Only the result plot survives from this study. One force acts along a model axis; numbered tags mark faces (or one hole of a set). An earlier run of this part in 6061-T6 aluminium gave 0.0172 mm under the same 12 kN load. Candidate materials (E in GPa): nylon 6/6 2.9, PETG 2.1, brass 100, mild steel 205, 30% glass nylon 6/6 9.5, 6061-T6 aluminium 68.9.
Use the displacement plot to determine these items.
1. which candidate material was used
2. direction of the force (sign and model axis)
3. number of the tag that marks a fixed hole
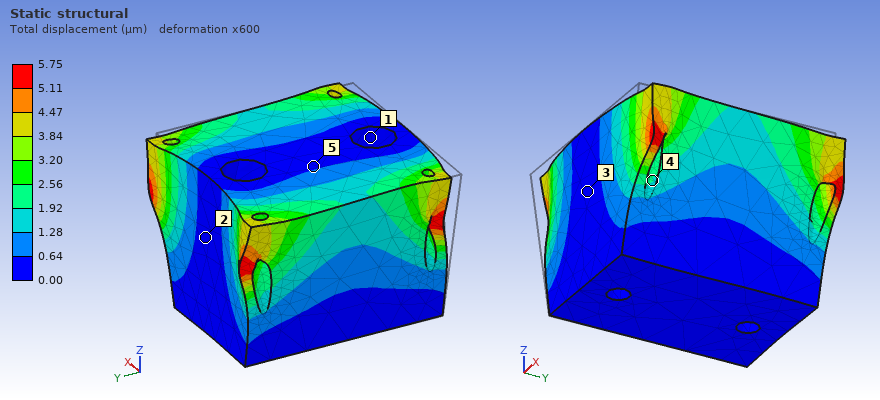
mild steel
+Y
1
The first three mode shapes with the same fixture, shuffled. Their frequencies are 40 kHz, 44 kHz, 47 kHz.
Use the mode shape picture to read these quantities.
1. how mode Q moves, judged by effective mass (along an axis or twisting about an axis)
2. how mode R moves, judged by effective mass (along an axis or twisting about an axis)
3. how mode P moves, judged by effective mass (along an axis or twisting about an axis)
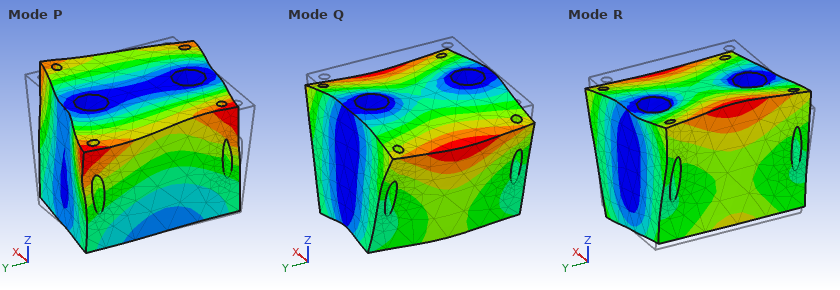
along Z
twisting about Y
twisting about Z
